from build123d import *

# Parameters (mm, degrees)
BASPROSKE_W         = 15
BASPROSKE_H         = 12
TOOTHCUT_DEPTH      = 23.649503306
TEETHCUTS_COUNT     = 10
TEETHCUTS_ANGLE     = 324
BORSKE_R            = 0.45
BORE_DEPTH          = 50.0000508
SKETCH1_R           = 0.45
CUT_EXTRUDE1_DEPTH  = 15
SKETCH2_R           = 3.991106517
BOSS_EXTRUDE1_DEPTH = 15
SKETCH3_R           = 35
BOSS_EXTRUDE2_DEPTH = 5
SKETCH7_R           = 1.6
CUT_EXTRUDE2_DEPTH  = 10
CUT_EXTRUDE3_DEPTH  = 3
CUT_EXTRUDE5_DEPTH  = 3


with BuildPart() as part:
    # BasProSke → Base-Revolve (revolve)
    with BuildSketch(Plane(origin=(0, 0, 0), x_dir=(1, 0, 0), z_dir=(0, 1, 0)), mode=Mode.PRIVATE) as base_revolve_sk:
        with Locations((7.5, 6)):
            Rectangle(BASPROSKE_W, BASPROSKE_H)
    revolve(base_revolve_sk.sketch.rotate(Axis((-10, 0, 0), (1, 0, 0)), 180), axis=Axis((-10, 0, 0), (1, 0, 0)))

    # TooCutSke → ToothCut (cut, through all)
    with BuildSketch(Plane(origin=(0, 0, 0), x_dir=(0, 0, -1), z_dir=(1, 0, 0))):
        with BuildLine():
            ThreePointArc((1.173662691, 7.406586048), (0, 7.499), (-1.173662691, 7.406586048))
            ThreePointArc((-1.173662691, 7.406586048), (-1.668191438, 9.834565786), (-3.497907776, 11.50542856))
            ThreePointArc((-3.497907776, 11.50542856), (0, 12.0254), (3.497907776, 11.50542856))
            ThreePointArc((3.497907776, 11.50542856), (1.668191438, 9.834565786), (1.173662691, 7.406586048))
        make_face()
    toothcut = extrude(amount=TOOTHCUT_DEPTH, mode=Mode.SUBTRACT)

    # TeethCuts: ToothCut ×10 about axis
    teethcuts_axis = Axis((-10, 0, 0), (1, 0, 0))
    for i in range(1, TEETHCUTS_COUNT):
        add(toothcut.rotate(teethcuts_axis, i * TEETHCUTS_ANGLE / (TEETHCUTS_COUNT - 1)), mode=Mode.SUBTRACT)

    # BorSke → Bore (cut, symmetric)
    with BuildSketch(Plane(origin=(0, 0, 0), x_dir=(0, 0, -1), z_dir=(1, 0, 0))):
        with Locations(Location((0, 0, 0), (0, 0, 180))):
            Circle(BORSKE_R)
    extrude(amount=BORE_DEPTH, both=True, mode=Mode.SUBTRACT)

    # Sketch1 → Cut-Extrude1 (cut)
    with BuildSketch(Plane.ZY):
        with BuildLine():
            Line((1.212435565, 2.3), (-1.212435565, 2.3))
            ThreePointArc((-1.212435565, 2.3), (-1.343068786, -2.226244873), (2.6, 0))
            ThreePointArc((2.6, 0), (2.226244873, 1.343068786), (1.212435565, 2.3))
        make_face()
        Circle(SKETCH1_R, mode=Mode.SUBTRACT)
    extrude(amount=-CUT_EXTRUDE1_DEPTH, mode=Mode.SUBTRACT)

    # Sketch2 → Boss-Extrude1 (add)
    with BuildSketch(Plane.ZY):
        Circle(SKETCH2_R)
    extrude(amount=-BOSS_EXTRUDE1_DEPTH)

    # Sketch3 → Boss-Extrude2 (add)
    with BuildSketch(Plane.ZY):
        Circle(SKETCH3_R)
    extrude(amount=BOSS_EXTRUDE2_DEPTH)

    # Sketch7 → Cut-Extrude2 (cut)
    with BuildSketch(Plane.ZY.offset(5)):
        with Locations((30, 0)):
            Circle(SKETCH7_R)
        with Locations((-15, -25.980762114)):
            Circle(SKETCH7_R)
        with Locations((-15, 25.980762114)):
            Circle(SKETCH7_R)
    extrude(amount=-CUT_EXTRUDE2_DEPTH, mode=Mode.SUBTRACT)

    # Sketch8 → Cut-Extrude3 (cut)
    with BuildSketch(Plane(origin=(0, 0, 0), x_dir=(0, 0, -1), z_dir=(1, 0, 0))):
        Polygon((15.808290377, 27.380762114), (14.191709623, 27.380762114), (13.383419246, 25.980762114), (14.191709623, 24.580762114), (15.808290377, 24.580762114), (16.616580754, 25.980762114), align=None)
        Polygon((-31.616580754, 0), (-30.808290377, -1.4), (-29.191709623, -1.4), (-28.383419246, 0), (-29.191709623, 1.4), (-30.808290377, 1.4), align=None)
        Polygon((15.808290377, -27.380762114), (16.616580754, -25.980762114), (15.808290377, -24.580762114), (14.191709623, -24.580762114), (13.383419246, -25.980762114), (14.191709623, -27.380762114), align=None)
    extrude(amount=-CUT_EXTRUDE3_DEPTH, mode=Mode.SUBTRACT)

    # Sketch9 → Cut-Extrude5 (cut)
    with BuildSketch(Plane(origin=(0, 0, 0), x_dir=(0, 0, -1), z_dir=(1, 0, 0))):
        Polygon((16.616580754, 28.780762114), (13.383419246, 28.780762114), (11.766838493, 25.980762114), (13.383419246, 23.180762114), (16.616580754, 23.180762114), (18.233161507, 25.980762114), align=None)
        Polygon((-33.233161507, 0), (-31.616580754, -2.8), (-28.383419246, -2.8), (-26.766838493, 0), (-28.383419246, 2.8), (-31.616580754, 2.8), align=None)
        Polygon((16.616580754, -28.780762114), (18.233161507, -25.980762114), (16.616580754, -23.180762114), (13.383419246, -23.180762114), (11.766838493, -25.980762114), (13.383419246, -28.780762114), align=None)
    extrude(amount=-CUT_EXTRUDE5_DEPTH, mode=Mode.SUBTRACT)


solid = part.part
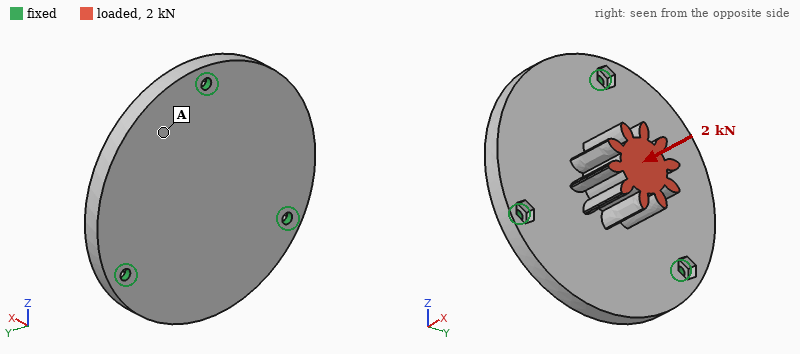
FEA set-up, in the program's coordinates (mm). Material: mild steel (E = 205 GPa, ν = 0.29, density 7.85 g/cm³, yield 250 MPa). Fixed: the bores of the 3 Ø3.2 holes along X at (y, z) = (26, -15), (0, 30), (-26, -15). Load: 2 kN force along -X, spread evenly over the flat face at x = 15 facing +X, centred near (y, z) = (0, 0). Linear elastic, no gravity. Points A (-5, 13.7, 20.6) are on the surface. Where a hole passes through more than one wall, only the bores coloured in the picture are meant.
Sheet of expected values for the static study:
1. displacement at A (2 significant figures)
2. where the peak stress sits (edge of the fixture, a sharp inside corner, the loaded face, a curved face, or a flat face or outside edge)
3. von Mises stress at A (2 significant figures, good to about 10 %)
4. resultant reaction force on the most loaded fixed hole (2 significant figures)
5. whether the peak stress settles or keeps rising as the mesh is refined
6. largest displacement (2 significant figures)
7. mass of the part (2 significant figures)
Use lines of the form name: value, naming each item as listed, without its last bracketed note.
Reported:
displacement at A: 10 µm
where the peak stress sits: edge of the fixture
von Mises stress at A: 20 MPa
resultant reaction force on the most loaded fixed hole: 1.1 kN
whether the peak stress settles or keeps rising as the mesh is refined: keeps rising
largest displacement: 20 µm
mass of the part: 180 g
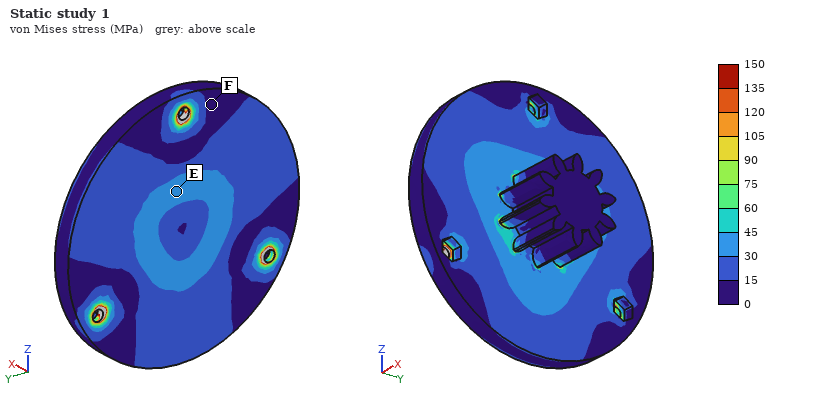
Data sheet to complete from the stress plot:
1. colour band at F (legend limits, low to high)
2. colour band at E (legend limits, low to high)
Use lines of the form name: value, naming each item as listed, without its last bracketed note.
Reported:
colour band at F: 0 to 15 MPa
colour band at E: 30 to 45 MPa
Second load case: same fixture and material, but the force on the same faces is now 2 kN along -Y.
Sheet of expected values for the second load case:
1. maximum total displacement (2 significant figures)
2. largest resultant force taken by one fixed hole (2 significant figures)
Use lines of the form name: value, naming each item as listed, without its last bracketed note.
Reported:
maximum total displacement: 29 µm
largest resultant force taken by one fixed hole: 1.4 kN
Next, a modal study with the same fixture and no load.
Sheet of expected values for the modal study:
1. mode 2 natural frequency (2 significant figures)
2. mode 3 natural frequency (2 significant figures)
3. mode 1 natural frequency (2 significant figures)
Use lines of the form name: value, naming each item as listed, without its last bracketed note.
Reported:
mode 2 natural frequency: 5100 Hz
mode 3 natural frequency: 5100 Hz
mode 1 natural frequency: 5100 Hz
